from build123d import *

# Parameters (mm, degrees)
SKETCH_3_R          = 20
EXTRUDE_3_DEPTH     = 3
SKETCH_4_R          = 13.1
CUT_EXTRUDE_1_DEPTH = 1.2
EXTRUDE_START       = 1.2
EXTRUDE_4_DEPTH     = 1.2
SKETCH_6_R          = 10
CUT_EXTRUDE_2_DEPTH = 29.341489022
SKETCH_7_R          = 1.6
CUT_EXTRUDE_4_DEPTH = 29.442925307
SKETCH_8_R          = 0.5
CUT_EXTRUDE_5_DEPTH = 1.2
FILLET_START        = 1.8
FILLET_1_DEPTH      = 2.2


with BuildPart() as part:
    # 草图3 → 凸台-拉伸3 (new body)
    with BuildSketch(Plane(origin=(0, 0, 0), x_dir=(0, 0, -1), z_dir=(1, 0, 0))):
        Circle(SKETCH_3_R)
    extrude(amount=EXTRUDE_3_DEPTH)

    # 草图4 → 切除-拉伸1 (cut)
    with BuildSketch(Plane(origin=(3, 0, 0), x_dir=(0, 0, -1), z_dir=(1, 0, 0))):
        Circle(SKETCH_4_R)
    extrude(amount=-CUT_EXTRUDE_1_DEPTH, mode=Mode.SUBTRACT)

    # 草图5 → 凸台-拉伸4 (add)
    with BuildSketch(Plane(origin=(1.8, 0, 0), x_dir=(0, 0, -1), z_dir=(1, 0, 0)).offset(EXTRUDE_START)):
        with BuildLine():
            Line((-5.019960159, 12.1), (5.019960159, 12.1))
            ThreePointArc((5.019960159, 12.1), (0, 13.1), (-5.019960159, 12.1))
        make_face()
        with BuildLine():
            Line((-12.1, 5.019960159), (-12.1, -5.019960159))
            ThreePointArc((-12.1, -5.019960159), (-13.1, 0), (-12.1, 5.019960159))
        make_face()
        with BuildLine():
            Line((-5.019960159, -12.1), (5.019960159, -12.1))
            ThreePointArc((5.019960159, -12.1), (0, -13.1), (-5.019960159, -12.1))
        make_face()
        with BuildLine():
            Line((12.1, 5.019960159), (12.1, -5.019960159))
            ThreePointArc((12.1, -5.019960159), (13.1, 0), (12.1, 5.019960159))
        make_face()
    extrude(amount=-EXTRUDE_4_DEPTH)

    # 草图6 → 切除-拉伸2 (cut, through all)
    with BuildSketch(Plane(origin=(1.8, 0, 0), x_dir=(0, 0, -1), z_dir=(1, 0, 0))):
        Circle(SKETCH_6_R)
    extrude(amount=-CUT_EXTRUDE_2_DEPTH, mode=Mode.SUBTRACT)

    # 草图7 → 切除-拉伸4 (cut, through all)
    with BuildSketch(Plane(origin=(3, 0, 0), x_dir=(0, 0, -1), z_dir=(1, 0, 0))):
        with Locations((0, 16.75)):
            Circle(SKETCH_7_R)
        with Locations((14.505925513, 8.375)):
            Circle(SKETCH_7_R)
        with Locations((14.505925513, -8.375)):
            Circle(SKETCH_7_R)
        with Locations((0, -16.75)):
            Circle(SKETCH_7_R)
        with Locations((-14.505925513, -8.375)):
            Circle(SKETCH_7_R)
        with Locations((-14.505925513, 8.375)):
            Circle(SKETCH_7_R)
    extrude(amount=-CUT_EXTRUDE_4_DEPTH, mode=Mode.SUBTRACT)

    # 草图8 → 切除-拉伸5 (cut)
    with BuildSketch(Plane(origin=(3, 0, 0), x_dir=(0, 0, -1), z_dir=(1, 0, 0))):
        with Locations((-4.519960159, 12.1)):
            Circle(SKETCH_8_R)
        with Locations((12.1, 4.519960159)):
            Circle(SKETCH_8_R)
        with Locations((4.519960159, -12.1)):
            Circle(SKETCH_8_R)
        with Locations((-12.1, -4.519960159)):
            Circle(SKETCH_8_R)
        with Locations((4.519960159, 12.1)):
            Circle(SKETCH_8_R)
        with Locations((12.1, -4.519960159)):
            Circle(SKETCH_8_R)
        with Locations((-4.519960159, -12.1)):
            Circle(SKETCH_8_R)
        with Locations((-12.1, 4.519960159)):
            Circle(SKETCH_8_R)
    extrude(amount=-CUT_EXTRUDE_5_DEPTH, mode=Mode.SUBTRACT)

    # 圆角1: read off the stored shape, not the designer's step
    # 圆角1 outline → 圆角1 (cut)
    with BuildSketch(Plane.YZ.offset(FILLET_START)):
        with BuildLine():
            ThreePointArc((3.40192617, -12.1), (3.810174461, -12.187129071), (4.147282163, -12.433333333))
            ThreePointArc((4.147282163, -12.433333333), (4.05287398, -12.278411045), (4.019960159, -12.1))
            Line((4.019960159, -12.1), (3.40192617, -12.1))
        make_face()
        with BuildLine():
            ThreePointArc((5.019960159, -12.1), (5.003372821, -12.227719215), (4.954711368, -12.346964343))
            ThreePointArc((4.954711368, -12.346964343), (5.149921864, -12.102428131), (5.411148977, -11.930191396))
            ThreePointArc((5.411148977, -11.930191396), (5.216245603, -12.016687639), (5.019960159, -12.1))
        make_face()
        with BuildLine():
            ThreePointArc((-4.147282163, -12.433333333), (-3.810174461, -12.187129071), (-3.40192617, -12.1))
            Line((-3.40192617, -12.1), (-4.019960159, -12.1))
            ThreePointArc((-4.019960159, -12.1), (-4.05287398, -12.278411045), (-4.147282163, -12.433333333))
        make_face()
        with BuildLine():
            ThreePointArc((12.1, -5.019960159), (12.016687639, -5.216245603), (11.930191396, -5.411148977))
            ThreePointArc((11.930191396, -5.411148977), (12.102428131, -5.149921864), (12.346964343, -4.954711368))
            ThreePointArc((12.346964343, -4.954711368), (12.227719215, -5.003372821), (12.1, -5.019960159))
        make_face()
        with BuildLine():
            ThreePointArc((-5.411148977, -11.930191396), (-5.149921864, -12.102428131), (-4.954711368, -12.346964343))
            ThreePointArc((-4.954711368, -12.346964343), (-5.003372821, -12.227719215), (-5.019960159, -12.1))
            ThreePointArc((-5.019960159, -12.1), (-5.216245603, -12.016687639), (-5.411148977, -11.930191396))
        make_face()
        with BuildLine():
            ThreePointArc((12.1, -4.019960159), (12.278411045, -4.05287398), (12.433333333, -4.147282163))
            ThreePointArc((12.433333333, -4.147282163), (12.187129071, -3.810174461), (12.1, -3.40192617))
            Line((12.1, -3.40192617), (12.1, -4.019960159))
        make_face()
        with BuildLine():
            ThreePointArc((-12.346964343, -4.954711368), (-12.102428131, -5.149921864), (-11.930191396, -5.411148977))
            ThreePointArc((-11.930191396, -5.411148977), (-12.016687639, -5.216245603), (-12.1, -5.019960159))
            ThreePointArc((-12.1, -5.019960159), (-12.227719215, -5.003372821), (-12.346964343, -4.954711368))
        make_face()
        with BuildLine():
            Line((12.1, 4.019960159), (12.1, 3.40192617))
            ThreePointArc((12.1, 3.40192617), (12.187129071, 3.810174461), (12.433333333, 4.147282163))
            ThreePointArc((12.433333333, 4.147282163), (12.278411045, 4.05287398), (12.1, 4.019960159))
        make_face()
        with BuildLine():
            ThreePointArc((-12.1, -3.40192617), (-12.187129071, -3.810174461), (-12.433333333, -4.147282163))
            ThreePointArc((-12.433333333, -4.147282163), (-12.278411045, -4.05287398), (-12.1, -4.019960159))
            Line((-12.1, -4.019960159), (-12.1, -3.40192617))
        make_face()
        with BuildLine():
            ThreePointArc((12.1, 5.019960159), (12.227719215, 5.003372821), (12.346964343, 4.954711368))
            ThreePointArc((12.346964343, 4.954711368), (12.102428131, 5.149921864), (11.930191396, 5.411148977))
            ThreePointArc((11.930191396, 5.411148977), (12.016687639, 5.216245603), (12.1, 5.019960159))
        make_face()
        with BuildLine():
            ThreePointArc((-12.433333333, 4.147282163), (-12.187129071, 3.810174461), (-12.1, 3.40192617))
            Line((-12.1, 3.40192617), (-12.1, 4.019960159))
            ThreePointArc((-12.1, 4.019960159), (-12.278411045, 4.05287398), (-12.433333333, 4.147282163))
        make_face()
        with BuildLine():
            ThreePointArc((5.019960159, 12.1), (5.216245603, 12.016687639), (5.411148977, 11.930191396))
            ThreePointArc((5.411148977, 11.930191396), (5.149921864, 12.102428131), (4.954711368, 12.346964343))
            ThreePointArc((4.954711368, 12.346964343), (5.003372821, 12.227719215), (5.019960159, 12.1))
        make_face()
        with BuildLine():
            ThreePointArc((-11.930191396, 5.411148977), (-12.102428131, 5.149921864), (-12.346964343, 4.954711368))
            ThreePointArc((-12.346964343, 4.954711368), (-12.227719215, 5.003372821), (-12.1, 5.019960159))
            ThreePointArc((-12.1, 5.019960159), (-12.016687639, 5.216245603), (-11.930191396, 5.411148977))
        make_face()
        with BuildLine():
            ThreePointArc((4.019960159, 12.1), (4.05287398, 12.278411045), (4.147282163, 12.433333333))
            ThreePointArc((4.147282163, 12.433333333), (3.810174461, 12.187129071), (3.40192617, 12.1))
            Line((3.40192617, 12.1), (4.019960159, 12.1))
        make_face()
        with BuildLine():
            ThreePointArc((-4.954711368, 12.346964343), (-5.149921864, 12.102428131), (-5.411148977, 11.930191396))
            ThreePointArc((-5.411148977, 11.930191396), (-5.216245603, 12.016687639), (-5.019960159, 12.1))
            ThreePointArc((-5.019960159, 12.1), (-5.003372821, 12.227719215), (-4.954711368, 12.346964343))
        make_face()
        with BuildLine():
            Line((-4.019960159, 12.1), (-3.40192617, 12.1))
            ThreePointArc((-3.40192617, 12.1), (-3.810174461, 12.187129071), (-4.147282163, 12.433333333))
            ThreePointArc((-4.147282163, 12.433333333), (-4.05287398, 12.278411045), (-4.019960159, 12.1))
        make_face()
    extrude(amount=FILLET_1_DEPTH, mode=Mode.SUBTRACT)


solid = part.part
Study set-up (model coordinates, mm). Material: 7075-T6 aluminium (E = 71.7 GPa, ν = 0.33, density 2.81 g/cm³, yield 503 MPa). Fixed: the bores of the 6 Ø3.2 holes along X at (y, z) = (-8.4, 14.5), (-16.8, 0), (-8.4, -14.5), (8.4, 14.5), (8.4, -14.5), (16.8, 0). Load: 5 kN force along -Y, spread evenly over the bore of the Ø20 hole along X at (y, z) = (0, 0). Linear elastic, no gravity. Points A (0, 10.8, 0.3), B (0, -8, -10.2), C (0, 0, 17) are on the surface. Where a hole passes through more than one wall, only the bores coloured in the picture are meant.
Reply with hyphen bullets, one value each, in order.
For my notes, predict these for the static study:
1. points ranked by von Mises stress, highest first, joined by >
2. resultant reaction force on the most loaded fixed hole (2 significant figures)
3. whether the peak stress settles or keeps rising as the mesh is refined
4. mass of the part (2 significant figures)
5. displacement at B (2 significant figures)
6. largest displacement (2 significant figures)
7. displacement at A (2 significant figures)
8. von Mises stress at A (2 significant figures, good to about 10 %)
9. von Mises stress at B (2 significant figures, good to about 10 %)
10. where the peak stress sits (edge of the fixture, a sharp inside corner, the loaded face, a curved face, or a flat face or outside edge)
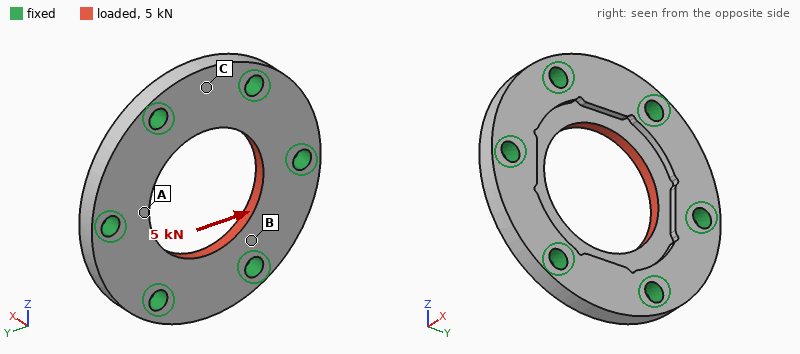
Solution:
- A > B > C
- 1.1 kN
- keeps rising
- 6.9 g
- 3.7 µm
- 8.5 µm
- 6.1 µm
- 53 MPa
- 33 MPa
- edge of the fixture
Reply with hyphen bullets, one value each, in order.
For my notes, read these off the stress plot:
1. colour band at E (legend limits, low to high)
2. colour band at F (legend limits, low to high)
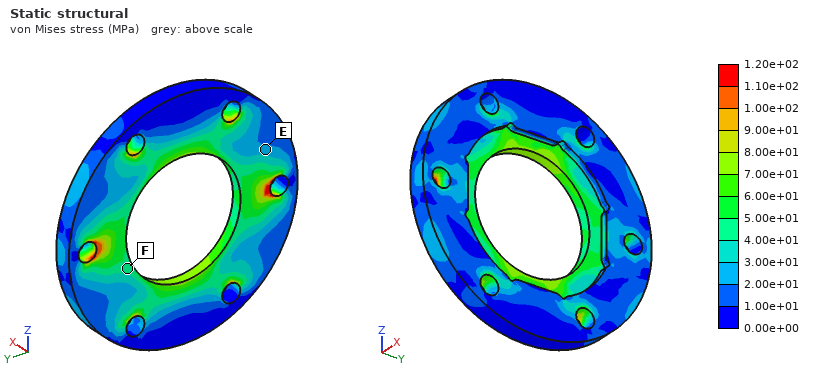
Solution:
- 2.00e+01 to 3.00e+01 MPa
- 4.00e+01 to 5.00e+01 MPa
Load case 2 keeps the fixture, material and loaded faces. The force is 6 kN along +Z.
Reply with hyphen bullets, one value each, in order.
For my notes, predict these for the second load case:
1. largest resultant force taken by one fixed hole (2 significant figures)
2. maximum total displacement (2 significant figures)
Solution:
- 1.2 kN
- 11 µm
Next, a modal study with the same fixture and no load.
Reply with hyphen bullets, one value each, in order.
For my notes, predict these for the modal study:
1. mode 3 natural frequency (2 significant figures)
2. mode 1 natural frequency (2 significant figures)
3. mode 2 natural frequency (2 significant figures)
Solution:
- 49 kHz
- 49 kHz
- 49 kHz
